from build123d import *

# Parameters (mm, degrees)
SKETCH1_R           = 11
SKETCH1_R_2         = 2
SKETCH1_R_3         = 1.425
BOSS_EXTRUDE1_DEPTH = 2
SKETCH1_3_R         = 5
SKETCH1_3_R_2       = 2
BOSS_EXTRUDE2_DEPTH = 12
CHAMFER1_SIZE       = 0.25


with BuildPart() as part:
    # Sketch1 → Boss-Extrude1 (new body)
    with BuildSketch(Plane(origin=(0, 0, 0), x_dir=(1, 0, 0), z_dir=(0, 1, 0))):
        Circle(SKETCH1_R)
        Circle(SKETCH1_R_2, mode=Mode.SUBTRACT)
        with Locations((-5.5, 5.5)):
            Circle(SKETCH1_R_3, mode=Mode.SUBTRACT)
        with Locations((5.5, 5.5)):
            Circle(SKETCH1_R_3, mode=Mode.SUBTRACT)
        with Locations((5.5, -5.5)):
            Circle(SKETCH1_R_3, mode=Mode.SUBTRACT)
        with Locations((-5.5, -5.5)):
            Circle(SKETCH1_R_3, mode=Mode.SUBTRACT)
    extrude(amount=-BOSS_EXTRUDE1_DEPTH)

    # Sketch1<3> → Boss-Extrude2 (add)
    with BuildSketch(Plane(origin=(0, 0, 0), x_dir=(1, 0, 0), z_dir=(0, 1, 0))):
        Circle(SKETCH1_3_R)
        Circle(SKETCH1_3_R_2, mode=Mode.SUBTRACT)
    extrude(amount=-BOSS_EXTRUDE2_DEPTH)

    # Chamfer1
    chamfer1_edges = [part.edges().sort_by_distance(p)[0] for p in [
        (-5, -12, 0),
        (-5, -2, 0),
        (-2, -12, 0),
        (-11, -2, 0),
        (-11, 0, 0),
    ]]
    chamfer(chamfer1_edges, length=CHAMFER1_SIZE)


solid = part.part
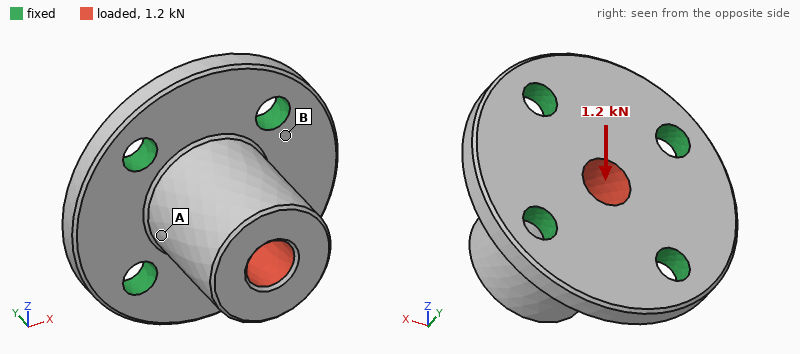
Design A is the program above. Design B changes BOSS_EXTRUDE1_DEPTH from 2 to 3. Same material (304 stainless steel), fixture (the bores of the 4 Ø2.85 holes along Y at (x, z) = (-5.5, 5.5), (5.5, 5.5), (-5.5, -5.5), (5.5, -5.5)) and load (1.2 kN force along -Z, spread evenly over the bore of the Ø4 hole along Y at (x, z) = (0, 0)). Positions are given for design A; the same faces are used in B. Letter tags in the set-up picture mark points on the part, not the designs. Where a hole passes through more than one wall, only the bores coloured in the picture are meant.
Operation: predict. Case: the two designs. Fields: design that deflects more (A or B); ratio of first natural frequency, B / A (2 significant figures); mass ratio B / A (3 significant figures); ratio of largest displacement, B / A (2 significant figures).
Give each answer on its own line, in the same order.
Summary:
A
1.3
1.21
0.58
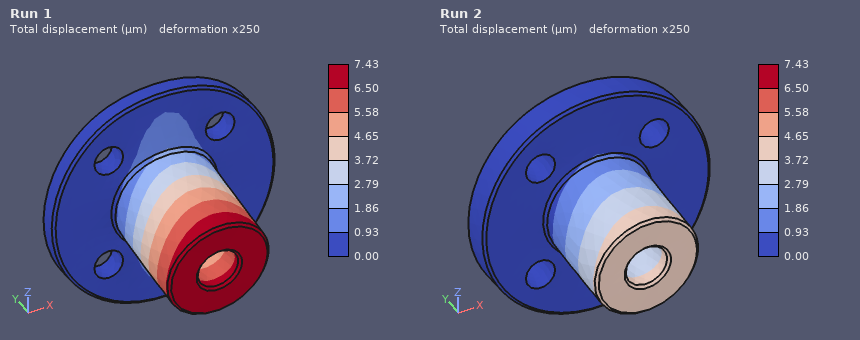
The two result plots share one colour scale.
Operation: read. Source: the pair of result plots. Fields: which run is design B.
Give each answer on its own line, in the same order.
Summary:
Run 2
